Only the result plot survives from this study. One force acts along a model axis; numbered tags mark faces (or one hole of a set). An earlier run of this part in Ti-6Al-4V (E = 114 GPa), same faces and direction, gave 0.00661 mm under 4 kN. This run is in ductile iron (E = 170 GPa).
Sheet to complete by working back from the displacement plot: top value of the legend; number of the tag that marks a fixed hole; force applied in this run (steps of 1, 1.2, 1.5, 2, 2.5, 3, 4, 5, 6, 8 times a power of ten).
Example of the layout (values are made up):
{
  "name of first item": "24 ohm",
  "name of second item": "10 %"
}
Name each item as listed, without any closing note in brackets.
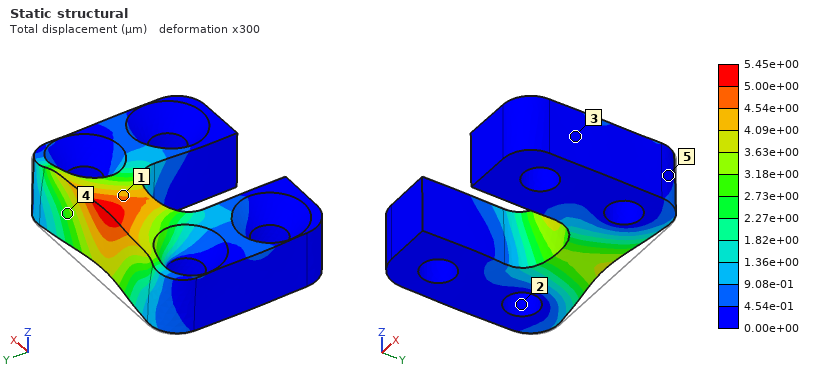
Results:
{
  "top value of the legend": "5.45e+00 µm",
  "number of the tag that marks a fixed hole": "2",
  "force applied in this run": "5 kN"
}
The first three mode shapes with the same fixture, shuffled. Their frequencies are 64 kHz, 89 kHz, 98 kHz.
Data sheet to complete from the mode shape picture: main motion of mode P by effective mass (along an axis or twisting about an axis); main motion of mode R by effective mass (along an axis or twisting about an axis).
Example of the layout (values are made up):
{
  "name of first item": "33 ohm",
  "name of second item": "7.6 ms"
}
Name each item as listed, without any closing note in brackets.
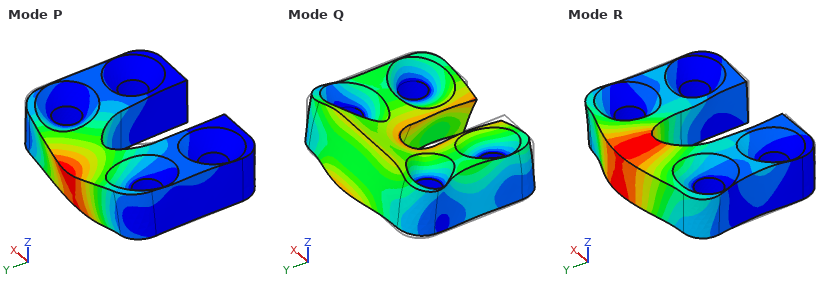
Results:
{
  "main motion of mode P by effective mass": "along Z",
  "main motion of mode R by effective mass": "along Y"
}
